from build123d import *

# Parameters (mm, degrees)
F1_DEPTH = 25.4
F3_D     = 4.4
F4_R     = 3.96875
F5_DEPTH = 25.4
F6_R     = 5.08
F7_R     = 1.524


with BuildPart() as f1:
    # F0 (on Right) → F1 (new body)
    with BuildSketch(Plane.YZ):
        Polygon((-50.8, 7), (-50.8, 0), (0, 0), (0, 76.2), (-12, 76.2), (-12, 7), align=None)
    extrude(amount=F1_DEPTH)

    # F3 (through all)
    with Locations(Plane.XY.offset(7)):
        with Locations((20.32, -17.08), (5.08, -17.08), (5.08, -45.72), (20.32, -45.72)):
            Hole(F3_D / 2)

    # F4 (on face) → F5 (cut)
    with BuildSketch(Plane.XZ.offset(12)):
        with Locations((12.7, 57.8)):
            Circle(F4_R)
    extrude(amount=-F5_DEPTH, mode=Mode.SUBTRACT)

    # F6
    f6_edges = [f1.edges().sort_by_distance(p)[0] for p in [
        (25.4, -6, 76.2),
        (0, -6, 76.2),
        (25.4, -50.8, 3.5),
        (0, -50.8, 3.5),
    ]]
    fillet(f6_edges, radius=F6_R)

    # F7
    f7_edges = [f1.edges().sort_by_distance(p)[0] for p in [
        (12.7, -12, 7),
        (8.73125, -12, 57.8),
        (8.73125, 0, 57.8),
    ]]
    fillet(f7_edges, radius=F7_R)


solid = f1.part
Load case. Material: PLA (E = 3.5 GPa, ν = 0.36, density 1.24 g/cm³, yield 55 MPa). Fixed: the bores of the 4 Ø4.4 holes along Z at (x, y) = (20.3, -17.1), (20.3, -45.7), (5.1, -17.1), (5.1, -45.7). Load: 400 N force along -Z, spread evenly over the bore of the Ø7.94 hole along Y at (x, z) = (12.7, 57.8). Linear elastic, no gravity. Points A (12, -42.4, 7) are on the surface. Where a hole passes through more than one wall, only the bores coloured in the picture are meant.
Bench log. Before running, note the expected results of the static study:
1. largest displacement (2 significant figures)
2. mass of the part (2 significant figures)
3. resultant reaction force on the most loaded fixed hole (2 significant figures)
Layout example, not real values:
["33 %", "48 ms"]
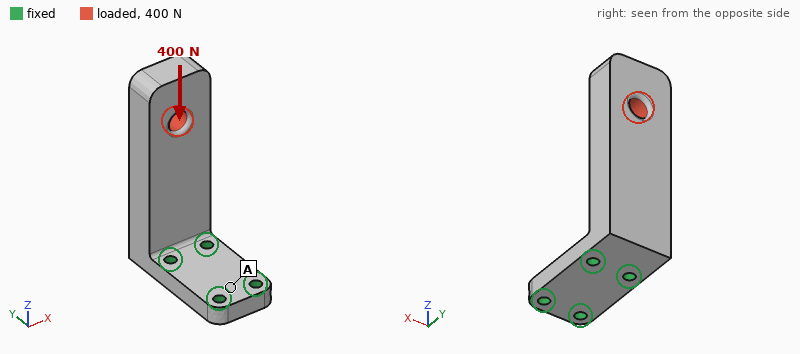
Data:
["0.60 mm", "36 g", "210 N"]
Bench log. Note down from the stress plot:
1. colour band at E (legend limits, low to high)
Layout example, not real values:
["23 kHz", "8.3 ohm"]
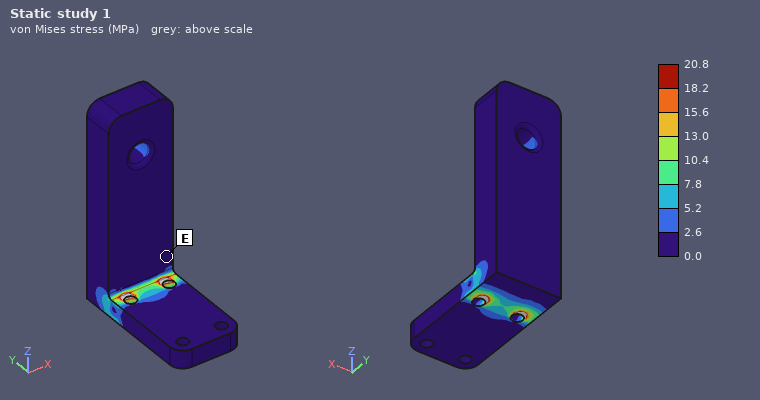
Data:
["0.0 to 2.6 MPa"]
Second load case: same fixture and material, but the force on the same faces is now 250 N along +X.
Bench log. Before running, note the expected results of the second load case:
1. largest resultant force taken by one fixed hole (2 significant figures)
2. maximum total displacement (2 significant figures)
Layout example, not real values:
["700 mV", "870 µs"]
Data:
["730 N", "1.1 mm"]
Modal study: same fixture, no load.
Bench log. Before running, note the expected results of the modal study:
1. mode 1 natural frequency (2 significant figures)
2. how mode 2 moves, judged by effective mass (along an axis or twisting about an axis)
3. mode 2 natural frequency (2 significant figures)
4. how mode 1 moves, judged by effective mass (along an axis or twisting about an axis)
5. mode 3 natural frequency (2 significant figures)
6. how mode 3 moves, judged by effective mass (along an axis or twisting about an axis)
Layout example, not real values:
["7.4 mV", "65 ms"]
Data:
["370 Hz", "along X", "720 Hz", "along Y", "2400 Hz", "along Z"]
